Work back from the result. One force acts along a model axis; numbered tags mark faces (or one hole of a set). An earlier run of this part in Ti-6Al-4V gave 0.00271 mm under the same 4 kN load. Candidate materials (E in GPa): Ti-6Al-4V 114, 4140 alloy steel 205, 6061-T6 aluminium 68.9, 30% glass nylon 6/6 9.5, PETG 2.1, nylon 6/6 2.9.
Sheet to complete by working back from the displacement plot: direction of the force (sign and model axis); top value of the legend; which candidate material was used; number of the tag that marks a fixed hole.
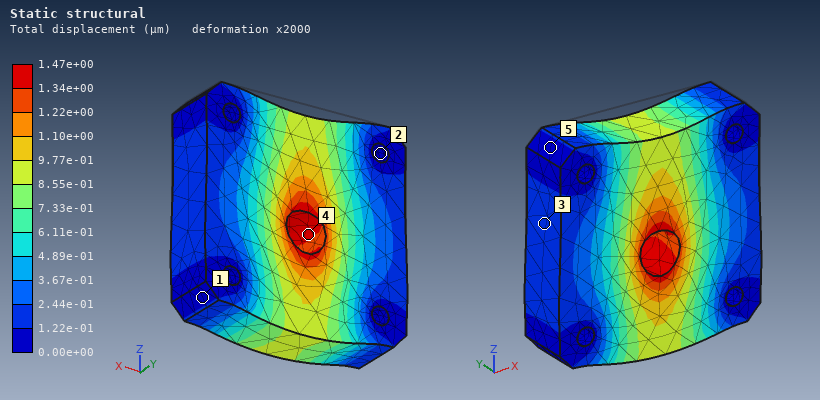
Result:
-Z
1.47e+00 µm
4140 alloy steel
2
